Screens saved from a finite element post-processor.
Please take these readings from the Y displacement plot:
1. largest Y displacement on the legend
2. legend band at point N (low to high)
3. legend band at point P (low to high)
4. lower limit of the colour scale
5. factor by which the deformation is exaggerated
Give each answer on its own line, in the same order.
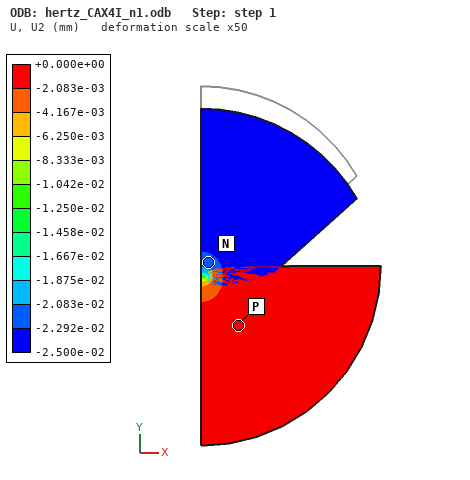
+0.000e+00 mm
-2.292e-02 to -2.083e-02 mm
-2.083e-03 to +0.000e+00 mm
-2.500e-02 mm
50
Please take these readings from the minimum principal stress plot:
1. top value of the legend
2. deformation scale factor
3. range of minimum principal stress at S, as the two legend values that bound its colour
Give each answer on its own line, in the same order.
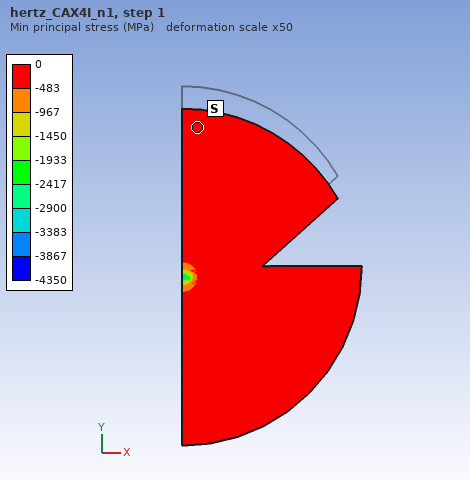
0 MPa
50
-483 to 0 MPa
